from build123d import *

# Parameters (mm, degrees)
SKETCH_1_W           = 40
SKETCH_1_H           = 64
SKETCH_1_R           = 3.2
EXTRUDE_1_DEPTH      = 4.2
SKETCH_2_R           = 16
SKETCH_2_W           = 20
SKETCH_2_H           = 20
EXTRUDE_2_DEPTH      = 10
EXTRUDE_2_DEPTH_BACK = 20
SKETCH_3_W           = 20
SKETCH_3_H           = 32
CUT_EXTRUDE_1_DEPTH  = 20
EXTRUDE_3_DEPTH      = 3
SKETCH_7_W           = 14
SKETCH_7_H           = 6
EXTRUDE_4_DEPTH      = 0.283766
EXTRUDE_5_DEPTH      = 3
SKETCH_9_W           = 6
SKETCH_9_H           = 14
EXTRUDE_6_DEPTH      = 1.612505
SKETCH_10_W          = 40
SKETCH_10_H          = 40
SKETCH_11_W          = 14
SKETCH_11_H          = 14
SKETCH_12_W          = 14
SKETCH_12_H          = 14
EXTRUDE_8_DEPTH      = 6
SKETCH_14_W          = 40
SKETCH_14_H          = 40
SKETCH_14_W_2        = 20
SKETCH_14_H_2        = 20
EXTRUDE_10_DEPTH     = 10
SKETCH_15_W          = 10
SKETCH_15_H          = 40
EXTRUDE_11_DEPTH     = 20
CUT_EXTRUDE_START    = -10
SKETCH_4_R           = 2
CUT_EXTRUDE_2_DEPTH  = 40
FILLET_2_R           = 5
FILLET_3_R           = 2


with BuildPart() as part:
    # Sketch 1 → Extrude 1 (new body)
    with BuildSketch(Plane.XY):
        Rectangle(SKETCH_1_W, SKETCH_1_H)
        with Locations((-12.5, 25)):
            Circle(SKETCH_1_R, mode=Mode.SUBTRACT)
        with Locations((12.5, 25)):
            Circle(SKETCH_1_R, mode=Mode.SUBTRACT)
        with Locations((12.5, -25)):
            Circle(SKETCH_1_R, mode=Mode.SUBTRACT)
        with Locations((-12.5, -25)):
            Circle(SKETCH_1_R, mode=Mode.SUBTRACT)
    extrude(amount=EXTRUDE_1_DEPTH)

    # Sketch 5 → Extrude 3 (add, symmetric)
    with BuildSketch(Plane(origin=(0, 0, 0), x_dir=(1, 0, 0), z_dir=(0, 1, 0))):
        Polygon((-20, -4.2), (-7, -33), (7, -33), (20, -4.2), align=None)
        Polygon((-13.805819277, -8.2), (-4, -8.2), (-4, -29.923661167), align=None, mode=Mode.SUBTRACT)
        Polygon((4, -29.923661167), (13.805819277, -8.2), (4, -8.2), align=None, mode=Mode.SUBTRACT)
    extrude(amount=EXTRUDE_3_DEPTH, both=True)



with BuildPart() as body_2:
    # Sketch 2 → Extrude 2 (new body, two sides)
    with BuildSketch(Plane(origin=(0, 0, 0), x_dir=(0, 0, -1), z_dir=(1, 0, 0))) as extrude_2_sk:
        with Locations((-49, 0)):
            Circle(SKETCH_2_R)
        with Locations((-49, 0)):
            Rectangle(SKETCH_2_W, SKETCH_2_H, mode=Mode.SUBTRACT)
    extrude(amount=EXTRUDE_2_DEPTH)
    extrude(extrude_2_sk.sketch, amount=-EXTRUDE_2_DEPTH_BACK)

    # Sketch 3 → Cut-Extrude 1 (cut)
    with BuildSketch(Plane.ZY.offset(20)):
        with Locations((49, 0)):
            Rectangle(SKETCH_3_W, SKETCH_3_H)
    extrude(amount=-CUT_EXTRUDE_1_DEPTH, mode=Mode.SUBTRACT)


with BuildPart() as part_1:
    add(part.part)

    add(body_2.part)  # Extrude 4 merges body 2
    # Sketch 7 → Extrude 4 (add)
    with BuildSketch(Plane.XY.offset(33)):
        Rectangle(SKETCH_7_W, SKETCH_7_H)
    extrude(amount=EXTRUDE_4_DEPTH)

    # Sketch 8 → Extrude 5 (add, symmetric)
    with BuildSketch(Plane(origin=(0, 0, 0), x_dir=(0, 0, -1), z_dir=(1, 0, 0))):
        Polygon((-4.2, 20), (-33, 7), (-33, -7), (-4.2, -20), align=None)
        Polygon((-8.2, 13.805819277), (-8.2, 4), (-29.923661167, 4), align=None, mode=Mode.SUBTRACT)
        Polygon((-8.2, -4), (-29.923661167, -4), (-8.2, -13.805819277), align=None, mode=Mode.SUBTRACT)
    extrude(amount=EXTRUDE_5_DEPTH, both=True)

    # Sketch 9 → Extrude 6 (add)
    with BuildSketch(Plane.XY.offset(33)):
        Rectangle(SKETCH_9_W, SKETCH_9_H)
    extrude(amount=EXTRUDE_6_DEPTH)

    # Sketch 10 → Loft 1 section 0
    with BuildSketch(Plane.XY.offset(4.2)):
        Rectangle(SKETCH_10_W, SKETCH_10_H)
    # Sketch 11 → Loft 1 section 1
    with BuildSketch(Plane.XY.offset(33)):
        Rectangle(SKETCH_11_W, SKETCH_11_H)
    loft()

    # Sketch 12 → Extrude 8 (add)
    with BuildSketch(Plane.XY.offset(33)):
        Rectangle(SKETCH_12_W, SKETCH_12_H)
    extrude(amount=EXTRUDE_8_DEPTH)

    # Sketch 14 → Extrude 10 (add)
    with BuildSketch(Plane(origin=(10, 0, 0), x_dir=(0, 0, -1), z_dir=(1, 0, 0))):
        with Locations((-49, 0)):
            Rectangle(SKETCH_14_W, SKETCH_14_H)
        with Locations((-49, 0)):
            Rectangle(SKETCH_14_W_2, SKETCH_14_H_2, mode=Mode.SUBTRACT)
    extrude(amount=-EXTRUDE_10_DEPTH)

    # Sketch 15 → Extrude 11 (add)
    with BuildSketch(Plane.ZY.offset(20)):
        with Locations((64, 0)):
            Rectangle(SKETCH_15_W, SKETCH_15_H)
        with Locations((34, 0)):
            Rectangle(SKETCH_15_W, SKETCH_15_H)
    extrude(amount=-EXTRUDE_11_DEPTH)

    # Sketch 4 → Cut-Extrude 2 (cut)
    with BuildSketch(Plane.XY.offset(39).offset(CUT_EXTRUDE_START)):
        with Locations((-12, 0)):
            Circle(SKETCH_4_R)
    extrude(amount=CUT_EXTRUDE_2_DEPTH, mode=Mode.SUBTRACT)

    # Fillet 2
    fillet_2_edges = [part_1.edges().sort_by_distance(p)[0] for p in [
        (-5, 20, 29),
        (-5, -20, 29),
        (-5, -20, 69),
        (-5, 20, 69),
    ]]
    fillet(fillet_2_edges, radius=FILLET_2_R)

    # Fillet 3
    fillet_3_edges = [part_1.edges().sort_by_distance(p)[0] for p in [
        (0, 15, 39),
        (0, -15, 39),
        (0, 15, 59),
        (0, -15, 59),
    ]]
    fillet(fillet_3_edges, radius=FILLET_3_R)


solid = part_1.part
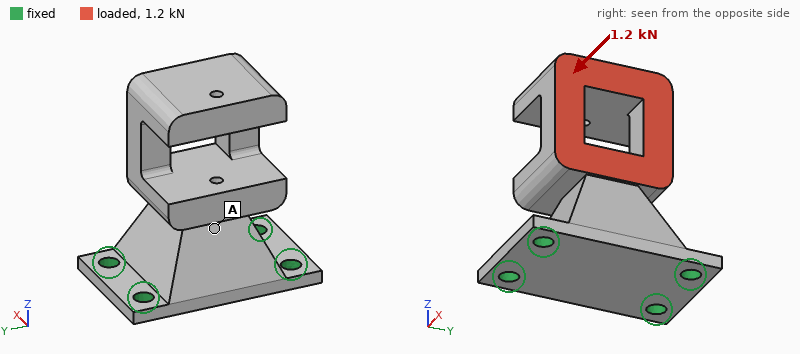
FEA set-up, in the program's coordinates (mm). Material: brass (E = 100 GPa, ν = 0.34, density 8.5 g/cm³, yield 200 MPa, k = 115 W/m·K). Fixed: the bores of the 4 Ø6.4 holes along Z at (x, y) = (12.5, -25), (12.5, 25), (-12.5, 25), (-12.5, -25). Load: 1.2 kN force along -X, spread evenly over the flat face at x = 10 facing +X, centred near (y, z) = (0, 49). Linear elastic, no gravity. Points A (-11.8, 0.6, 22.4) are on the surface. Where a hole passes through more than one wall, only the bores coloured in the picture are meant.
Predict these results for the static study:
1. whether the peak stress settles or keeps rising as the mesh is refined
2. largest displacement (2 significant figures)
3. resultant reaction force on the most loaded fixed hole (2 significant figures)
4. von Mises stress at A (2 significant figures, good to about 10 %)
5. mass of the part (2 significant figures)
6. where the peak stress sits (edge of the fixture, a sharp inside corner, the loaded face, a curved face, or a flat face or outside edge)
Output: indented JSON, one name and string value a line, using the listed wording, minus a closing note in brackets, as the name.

{
  "whether the peak stress settles or keeps rising as the mesh is refined": "keeps rising",
  "largest displacement": "0.10 mm",
  "resultant reaction force on the most loaded fixed hole": "1.3 kN",
  "von Mises stress at A": "13 MPa",
  "mass of the part": "500 g",
  "where the peak stress sits": "edge of the fixture"
}
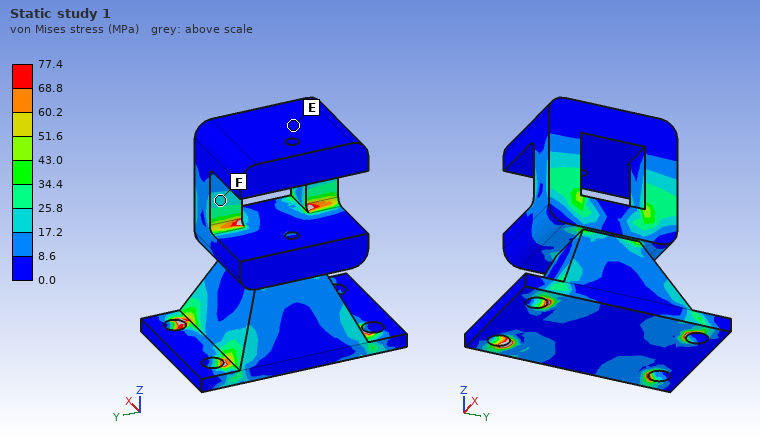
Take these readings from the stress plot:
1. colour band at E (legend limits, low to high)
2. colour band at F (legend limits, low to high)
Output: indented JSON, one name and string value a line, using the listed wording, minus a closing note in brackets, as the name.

{
  "colour band at E": "0.0 to 8.6 MPa",
  "colour band at F": "17.2 to 25.8 MPa"
}
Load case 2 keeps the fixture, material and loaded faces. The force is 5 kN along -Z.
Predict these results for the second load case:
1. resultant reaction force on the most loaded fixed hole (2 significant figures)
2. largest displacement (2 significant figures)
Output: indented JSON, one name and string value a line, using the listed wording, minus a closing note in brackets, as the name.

{
  "resultant reaction force on the most loaded fixed hole": "2.6 kN",
  "largest displacement": "0.13 mm"
}
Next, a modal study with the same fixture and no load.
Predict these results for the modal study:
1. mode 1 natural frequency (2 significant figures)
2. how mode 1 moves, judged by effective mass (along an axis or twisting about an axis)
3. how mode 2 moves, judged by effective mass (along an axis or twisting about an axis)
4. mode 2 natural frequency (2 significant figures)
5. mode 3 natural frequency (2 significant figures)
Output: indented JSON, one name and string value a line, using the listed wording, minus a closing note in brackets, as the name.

{
  "mode 1 natural frequency": "1300 Hz",
  "how mode 1 moves, judged by effective mass": "along X",
  "how mode 2 moves, judged by effective mass": "along Y",
  "mode 2 natural frequency": "1800 Hz",
  "mode 3 natural frequency": "3300 Hz"
}
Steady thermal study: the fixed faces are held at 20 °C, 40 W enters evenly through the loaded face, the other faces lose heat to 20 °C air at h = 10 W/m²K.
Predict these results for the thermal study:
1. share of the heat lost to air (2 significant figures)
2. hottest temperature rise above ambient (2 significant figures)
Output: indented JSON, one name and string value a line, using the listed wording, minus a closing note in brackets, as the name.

{
  "share of the heat lost to air": "8.3 %",
  "hottest temperature rise above ambient": "52 K"
}
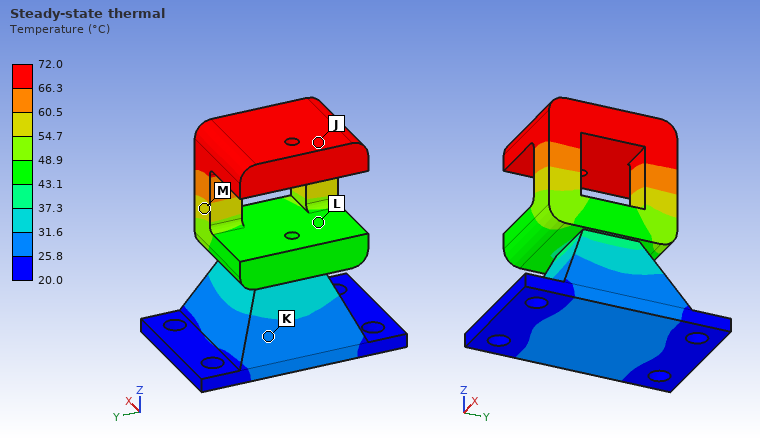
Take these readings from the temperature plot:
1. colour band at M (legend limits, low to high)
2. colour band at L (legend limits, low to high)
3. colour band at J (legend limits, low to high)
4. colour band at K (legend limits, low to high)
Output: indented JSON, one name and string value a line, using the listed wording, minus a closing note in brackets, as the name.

{
  "colour band at M": "54.7 to 60.5 °C",
  "colour band at L": "43.1 to 48.9 °C",
  "colour band at J": "66.3 to 72.0 °C",
  "colour band at K": "25.8 to 31.6 °C"
}
